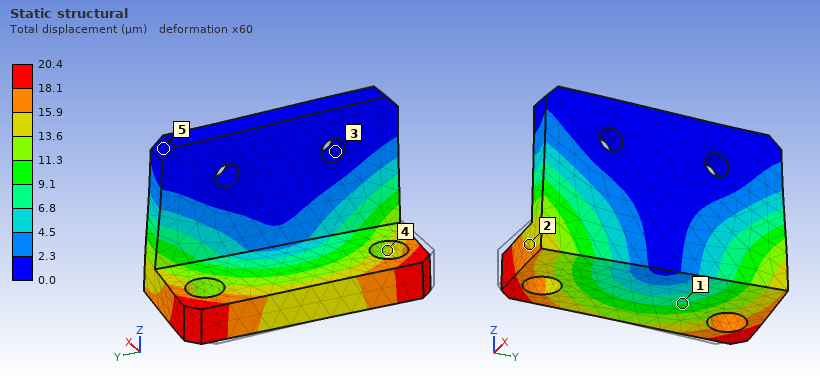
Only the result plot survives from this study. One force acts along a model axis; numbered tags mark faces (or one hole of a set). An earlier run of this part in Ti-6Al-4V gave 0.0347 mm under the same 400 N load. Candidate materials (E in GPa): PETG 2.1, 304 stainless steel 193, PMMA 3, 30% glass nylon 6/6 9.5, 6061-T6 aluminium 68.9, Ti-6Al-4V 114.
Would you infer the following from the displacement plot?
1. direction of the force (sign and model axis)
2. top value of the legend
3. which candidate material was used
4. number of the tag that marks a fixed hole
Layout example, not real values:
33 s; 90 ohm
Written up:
+Y; 20.4 µm; 304 stainless steel; 3
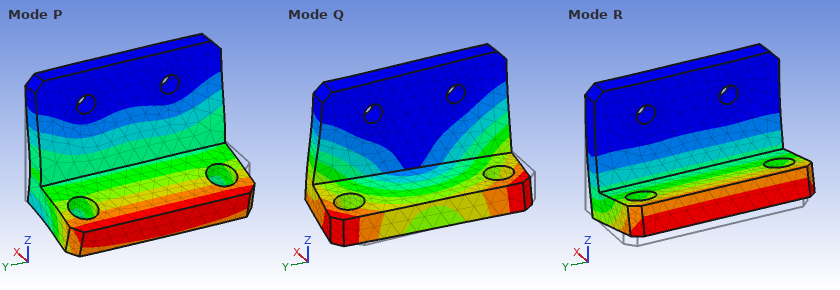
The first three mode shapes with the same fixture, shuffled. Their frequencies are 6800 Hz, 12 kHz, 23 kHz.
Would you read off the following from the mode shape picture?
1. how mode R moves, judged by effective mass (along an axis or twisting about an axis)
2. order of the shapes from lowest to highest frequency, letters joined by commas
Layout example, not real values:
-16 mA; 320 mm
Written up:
along X; R, Q, P
